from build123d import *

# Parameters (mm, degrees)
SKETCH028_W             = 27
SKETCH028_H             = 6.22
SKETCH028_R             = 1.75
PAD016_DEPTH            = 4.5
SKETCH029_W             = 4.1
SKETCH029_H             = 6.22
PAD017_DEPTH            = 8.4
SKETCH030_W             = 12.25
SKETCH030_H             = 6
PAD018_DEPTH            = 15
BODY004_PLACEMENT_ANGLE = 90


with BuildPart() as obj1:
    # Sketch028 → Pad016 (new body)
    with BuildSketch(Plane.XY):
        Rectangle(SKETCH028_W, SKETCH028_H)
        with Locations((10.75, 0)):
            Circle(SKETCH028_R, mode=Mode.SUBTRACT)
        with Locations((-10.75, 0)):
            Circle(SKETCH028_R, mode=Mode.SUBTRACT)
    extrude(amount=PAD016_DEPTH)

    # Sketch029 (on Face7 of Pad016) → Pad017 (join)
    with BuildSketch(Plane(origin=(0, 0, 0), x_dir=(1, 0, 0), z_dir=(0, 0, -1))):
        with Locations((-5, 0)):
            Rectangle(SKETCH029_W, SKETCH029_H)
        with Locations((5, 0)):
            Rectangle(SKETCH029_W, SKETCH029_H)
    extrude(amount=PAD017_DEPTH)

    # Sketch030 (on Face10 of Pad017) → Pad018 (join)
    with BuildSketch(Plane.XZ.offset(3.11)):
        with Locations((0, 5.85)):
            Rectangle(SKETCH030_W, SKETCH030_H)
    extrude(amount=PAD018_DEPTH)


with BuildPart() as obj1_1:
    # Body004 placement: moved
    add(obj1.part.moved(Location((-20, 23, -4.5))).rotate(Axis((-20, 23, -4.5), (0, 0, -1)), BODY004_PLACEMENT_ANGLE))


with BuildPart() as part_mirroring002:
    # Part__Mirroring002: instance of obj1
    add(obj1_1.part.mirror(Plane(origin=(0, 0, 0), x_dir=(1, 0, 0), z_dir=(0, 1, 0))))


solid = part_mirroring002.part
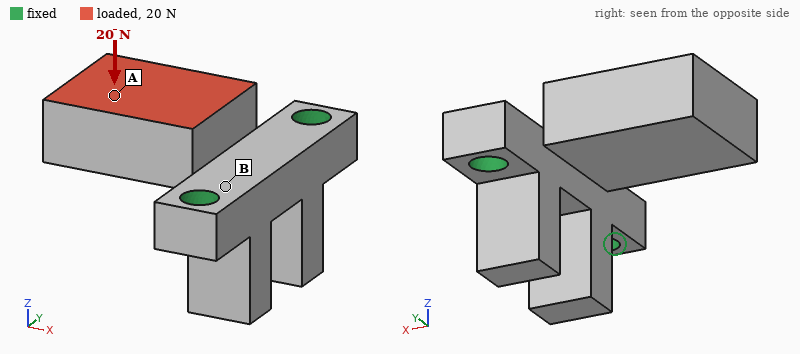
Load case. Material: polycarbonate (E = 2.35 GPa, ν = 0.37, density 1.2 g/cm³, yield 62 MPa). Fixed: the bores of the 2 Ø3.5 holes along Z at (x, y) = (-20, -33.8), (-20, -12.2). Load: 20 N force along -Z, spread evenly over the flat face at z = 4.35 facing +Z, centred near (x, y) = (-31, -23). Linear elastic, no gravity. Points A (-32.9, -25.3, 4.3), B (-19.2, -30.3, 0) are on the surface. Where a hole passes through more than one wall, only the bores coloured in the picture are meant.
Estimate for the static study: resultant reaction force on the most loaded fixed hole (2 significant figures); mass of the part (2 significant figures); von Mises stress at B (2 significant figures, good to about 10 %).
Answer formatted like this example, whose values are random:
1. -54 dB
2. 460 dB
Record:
1. 10 N
2. 2.6 g
3. 4.4 MPa
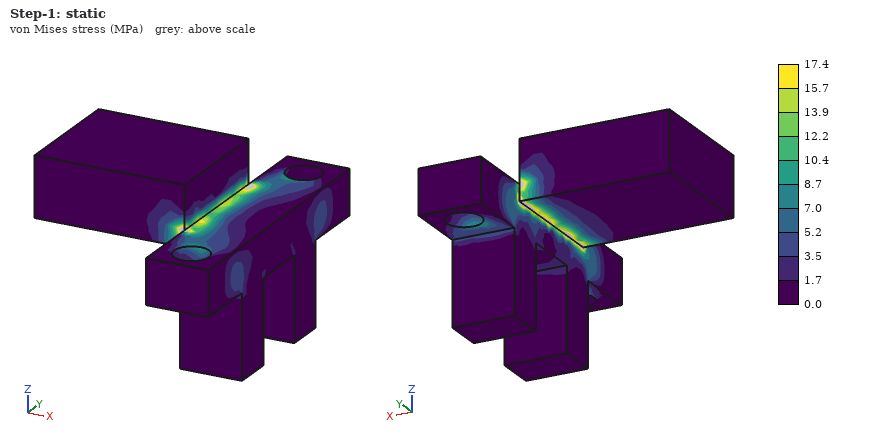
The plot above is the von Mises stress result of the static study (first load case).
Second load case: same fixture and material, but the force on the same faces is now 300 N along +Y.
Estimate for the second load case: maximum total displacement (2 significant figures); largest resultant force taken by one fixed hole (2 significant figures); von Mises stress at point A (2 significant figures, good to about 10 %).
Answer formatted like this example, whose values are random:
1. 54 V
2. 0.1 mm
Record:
1. 0.46 mm
2. 260 N
3. 8.7 MPa
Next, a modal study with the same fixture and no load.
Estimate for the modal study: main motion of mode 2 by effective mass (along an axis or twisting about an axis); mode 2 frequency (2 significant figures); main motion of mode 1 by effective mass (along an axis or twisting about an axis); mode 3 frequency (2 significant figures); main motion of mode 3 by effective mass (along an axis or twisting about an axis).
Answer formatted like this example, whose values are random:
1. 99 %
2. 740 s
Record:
1. along Y
2. 4200 Hz
3. along Z
4. 6100 Hz
5. along X
